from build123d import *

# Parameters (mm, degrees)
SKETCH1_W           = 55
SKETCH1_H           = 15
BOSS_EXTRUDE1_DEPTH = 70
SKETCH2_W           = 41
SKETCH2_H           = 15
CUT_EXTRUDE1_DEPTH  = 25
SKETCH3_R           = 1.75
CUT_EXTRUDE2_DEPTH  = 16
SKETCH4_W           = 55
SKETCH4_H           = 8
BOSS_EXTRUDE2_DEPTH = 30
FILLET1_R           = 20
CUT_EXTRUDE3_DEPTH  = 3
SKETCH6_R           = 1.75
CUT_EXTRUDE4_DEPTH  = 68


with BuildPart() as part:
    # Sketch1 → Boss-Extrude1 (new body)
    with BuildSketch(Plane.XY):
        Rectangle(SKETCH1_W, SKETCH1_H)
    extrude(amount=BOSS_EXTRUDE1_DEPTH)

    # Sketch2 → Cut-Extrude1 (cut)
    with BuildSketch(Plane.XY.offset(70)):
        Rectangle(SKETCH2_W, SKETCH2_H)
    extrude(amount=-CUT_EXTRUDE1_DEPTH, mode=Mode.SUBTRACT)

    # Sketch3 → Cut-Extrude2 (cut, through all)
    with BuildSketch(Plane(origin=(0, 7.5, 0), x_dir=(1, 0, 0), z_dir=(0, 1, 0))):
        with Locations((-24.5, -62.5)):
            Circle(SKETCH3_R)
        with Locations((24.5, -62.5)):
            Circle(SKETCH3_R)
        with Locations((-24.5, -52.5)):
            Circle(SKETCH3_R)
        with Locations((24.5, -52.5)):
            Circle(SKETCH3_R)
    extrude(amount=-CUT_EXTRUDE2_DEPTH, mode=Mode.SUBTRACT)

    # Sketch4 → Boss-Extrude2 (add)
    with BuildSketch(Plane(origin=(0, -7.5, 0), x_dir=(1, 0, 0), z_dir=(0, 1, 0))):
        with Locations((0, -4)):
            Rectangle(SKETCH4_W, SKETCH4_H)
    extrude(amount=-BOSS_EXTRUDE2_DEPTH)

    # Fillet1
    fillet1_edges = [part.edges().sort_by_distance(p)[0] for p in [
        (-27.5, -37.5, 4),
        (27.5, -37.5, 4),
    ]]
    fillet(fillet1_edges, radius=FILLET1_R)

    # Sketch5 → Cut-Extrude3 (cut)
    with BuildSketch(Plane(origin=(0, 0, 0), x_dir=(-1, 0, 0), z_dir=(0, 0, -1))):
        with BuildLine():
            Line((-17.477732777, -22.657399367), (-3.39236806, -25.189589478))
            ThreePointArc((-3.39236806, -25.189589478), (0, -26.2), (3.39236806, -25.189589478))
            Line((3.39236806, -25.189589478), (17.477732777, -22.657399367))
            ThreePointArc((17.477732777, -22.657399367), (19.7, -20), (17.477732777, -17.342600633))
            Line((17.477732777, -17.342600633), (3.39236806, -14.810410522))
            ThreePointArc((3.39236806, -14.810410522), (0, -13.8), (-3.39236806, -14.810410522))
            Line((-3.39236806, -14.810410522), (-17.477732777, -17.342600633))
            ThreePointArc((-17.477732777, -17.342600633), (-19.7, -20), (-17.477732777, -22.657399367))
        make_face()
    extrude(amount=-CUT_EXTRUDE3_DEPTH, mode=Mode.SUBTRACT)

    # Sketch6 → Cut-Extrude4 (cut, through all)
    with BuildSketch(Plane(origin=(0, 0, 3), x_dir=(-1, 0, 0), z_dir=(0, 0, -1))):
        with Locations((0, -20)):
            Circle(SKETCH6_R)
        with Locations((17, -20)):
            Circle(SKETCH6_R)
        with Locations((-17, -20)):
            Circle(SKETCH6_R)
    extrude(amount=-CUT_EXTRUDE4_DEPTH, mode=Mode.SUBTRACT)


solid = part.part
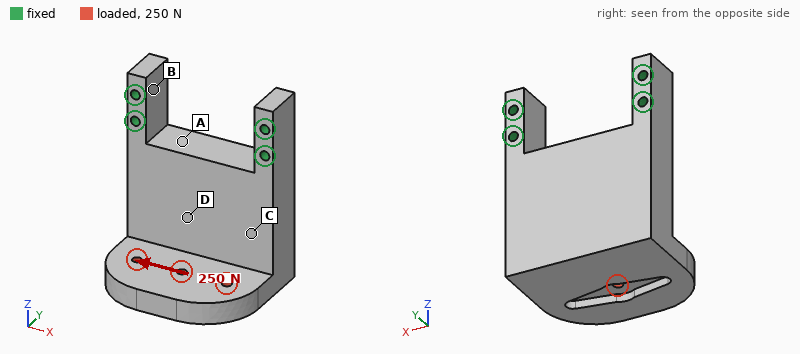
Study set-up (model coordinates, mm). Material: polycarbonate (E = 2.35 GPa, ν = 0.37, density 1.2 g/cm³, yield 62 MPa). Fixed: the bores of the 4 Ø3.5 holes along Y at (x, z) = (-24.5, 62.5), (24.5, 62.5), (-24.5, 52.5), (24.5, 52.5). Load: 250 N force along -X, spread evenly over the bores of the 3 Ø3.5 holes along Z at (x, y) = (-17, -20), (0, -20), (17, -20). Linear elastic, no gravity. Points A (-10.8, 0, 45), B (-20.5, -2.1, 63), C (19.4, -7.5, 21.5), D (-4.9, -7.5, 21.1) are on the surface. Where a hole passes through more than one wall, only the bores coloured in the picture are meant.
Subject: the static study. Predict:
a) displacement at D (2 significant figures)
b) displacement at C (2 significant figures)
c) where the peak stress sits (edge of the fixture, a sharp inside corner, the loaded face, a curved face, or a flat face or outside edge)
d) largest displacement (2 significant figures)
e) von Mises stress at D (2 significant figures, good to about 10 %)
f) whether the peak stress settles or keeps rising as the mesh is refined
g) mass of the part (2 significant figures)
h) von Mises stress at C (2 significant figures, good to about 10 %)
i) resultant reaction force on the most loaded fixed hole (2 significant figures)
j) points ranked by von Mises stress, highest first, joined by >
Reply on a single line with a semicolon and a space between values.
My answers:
0.068 mm; 0.089 mm; edge of the fixture; 0.26 mm; 3.0 MPa; keeps rising; 63 g; 2.4 MPa; 280 N; D > C > A > B
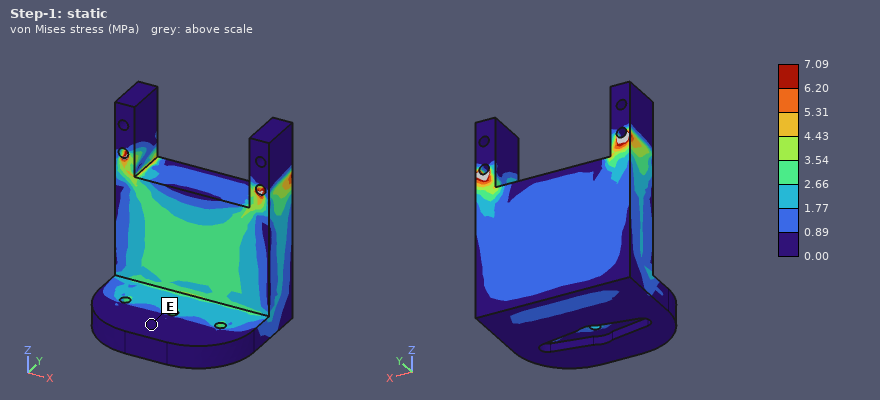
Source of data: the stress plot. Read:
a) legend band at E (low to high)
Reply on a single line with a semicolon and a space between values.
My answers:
0.00 to 0.89 MPa
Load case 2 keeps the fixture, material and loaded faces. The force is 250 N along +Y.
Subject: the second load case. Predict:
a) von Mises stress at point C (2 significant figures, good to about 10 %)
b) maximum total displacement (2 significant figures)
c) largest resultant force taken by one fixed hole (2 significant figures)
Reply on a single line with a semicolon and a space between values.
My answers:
2.3 MPa; 1.1 mm; 140 N
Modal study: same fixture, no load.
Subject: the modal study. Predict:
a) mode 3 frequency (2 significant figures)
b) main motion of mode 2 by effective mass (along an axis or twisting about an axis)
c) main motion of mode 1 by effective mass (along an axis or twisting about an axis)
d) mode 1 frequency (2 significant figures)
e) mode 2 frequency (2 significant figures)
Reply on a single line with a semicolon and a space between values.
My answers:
1500 Hz; along X; along Y; 480 Hz; 1200 Hz
